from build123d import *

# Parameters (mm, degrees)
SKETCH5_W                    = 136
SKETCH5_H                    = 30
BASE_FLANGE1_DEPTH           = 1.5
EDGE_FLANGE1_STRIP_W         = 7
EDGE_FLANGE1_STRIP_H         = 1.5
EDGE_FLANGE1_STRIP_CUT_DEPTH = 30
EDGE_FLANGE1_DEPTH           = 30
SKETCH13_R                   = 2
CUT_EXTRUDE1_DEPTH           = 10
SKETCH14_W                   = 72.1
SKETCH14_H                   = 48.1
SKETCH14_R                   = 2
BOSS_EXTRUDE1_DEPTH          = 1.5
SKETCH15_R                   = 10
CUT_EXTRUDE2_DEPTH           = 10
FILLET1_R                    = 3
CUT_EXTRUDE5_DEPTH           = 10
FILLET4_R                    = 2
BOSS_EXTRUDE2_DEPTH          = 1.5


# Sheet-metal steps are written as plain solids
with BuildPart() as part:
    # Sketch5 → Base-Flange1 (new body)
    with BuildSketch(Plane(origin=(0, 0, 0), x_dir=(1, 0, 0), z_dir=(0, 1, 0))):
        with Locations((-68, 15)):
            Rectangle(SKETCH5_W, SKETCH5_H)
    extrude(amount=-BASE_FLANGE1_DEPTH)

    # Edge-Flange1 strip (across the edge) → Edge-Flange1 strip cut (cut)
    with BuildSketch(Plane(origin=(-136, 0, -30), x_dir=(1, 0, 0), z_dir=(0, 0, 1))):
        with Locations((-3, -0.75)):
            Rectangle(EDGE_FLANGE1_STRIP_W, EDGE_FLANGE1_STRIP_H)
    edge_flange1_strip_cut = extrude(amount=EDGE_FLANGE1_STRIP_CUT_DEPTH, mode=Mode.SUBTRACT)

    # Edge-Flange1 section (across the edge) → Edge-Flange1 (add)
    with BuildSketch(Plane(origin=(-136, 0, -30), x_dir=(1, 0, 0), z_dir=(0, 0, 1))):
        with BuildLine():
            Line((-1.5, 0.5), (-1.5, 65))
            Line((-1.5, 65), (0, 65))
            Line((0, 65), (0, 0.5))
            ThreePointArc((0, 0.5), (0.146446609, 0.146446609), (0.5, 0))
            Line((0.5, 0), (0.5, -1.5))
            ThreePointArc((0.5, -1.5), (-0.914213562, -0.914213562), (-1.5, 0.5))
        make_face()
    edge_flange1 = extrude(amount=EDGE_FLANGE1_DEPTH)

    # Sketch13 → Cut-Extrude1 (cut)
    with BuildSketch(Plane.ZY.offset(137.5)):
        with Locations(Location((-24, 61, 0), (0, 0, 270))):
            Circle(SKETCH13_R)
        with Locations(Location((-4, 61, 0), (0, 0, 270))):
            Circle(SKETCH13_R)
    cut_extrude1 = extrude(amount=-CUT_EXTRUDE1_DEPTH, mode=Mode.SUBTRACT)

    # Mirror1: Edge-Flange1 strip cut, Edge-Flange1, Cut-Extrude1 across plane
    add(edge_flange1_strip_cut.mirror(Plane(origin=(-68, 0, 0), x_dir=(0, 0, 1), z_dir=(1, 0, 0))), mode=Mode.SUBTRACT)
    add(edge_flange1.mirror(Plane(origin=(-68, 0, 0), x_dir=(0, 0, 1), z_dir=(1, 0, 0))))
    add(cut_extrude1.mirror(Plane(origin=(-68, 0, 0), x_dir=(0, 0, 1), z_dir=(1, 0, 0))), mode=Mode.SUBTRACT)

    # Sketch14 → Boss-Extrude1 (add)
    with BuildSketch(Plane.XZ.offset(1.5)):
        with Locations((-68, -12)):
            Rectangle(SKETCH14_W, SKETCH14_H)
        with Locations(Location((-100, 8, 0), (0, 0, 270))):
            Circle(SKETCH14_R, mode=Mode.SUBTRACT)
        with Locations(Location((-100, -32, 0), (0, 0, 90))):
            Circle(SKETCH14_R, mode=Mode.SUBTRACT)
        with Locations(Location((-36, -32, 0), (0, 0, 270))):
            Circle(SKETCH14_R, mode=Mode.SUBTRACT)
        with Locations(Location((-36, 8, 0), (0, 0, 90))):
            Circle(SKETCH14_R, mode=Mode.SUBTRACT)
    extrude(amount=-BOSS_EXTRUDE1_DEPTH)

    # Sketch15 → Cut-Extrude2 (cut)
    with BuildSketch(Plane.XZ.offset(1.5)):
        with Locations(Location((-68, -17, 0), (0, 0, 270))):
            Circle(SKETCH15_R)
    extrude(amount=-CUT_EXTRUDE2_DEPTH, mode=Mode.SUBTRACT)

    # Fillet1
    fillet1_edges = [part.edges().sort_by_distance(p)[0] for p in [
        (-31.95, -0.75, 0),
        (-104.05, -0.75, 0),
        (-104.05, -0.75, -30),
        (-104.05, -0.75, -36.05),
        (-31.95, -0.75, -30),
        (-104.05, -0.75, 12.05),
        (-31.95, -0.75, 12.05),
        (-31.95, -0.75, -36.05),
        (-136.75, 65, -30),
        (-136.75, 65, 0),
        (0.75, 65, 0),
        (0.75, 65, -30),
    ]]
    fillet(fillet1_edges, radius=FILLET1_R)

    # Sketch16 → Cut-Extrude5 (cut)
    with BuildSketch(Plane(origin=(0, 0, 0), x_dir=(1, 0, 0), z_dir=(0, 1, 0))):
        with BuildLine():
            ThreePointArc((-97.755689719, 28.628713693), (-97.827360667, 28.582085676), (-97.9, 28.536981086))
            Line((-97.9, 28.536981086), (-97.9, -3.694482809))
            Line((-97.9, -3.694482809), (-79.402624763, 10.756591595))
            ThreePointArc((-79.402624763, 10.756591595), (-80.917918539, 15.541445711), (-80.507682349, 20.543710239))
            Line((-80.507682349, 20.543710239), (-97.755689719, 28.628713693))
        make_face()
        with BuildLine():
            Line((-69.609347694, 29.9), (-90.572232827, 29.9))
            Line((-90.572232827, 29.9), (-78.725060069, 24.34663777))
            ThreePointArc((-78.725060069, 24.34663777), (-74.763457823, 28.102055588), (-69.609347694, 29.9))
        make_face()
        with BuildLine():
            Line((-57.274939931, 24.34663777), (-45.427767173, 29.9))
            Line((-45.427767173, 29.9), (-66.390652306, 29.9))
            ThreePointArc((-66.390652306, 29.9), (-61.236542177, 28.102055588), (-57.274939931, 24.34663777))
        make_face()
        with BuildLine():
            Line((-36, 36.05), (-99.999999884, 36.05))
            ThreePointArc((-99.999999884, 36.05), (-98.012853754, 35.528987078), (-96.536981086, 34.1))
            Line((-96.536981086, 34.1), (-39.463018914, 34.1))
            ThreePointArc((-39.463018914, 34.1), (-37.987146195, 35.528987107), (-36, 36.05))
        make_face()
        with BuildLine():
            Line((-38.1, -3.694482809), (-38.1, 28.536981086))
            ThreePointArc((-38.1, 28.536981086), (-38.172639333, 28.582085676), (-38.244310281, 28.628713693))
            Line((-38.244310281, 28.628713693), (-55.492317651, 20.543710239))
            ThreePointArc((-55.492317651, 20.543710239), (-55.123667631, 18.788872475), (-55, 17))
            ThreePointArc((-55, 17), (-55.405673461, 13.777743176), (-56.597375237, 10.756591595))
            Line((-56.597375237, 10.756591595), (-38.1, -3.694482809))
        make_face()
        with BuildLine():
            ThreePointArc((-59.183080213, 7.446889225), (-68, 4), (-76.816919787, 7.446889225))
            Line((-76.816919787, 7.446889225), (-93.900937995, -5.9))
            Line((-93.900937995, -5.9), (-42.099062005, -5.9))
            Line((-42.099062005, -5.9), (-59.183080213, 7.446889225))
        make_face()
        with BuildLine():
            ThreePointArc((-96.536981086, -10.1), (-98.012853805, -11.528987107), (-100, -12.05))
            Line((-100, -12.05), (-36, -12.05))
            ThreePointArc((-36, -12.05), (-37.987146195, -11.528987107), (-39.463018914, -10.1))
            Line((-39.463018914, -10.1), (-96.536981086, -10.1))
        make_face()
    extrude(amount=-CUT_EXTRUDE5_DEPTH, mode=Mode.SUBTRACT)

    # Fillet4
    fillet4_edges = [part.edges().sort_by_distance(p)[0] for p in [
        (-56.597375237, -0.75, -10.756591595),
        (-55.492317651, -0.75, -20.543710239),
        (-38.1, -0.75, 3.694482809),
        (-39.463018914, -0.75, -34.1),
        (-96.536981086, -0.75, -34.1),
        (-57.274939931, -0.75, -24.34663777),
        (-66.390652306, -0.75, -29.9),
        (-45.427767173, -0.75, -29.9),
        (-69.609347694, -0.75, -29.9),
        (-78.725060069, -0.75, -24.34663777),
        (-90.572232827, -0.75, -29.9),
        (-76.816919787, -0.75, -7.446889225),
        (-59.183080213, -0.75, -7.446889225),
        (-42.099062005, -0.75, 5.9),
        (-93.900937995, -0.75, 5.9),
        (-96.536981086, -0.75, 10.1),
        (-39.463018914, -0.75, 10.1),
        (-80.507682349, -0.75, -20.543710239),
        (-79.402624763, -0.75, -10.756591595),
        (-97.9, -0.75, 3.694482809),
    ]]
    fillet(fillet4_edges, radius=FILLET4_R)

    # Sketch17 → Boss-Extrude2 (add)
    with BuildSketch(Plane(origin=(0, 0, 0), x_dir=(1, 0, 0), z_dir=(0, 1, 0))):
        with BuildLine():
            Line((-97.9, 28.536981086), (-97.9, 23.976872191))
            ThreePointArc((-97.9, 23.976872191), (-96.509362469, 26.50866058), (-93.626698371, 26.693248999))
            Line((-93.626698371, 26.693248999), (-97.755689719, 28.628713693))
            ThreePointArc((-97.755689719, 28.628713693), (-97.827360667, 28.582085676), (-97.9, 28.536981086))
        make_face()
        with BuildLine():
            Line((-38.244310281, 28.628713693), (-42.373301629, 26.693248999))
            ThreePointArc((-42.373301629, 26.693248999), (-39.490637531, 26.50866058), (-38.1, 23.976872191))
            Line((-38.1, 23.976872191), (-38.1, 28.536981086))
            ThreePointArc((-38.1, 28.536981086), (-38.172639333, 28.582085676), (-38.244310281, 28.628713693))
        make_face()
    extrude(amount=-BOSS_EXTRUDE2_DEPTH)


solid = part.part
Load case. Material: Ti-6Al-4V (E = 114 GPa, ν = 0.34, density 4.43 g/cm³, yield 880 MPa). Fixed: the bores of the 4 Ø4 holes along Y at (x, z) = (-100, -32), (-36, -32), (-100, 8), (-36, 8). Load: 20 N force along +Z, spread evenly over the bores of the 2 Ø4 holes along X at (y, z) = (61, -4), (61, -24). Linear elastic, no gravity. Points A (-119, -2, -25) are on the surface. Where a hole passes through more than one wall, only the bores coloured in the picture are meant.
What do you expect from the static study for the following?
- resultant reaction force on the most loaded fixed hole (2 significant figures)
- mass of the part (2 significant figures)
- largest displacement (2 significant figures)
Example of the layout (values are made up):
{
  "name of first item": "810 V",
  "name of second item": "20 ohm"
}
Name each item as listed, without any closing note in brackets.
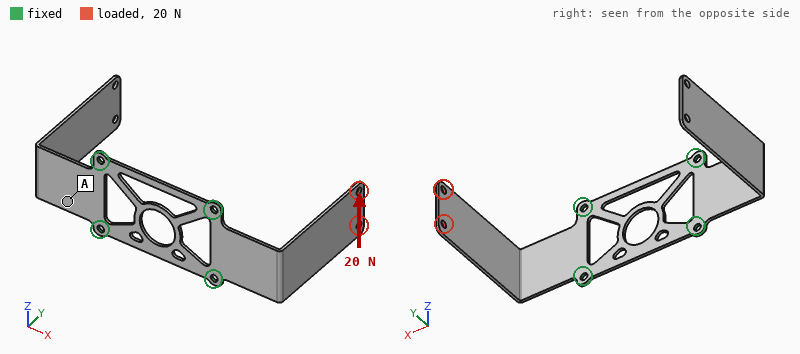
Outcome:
{
  "resultant reaction force on the most loaded fixed hole": "46 N",
  "mass of the part": "50 g",
  "largest displacement": "1.6 mm"
}
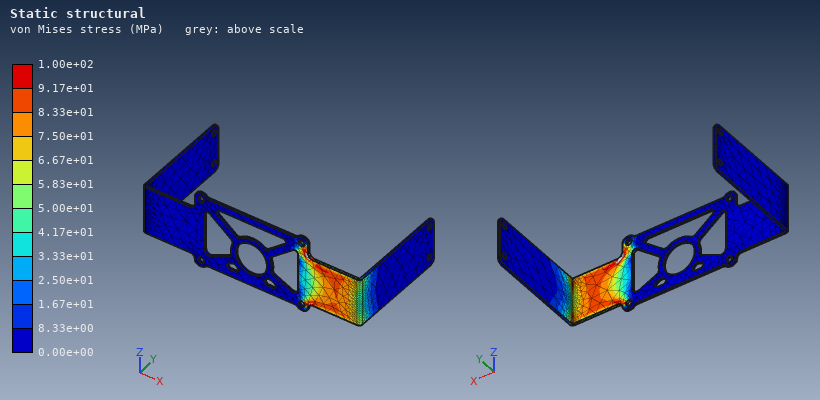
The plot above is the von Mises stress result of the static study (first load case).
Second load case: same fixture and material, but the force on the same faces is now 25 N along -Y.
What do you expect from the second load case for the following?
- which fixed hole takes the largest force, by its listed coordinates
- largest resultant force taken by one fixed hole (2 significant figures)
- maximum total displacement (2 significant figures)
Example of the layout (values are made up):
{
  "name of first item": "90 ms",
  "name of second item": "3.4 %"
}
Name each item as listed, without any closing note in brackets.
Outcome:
{
  "which fixed hole takes the largest force, by its listed coordinates": "(-36, -32)",
  "largest resultant force taken by one fixed hole": "14 N",
  "maximum total displacement": "1.7 mm"
}
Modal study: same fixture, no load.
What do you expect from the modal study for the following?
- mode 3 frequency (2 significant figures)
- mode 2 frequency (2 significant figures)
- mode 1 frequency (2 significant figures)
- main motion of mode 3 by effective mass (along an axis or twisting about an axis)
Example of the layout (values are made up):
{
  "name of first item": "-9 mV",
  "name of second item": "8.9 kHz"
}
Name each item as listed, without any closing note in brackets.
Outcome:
{
  "mode 3 frequency": "270 Hz",
  "mode 2 frequency": "140 Hz",
  "mode 1 frequency": "140 Hz",
  "main motion of mode 3 by effective mass": "along Z"
}
